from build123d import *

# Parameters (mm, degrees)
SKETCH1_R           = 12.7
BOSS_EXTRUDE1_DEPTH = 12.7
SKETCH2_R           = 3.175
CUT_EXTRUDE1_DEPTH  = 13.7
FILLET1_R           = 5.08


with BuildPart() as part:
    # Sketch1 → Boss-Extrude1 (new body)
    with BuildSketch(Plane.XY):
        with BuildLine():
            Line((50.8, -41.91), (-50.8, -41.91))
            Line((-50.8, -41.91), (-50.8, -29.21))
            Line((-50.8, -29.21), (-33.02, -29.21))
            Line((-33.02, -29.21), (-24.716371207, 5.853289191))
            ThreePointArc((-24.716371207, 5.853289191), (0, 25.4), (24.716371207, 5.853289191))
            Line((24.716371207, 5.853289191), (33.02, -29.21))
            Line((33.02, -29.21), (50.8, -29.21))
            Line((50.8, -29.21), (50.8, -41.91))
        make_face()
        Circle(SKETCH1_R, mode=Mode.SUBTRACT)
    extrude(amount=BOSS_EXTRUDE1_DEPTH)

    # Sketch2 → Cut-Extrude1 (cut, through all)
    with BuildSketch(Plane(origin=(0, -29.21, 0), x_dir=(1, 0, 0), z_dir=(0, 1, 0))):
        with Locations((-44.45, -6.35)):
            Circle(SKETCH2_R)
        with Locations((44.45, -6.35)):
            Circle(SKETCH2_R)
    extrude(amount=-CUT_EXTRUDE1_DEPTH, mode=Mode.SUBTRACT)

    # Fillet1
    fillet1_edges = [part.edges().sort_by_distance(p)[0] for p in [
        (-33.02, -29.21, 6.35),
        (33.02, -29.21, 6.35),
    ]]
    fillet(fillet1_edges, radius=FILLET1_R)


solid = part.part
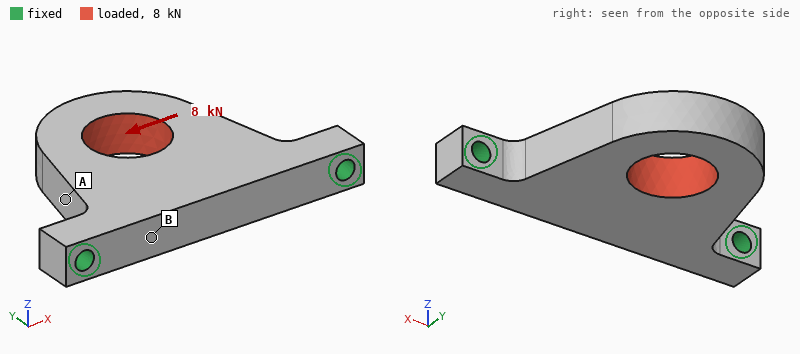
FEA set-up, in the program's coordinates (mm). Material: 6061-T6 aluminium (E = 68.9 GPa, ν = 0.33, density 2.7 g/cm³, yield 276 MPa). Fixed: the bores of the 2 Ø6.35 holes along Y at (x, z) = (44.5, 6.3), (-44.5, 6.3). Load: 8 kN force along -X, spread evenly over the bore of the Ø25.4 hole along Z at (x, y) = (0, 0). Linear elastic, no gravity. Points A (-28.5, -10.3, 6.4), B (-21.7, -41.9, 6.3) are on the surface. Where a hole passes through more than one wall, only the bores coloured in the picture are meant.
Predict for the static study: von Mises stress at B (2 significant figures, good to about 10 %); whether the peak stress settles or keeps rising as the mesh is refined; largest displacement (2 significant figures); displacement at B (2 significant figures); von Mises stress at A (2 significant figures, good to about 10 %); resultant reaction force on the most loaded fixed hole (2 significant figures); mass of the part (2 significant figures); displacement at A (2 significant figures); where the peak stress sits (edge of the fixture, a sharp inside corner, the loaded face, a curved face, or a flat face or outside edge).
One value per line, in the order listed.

12 MPa
keeps rising
73 µm
12 µm
36 MPa
5.5 kN
120 g
35 µm
edge of the fixture
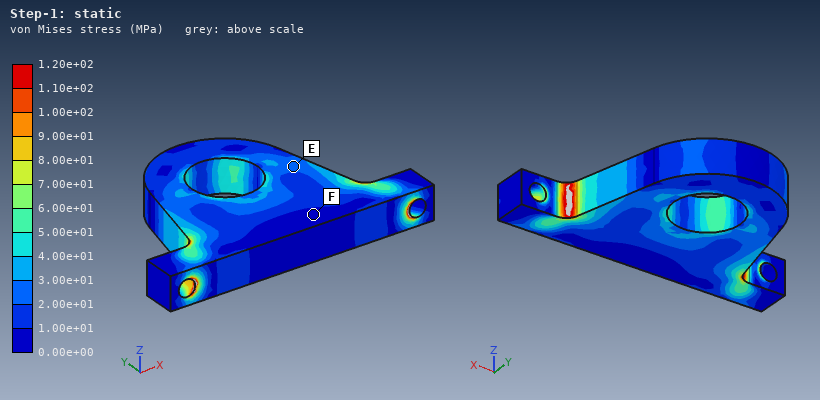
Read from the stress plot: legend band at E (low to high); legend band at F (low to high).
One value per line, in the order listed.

2.00e+01 to 3.00e+01 MPa
0.00e+00 to 1.00e+01 MPa
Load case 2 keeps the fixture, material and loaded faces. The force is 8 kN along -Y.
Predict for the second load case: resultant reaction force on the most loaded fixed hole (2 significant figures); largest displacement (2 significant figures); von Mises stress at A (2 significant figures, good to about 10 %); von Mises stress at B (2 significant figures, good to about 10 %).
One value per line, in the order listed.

4.6 kN
37 µm
21 MPa
20 MPa
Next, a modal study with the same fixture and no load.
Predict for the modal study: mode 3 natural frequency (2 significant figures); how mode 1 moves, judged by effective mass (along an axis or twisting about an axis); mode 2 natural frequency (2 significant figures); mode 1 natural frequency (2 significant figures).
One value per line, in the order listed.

6800 Hz
along Z
6600 Hz
1700 Hz
